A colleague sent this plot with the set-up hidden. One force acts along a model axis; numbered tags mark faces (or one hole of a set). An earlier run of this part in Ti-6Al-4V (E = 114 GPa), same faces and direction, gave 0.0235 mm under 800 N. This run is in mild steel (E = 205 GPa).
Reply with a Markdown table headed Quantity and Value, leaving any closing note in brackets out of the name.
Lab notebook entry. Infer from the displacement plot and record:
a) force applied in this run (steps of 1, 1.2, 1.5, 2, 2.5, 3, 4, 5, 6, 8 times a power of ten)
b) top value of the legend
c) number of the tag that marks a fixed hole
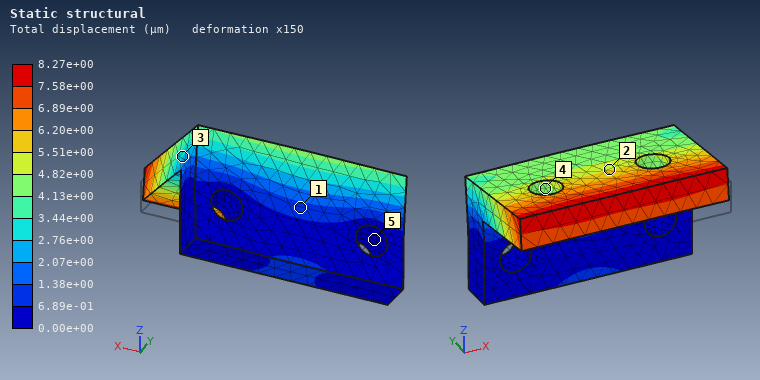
| Quantity | Value |
|---|---|
| force applied in this run | 500 N |
| top value of the legend | 8.27e+00 µm |
| number of the tag that marks a fixed hole | 5 |
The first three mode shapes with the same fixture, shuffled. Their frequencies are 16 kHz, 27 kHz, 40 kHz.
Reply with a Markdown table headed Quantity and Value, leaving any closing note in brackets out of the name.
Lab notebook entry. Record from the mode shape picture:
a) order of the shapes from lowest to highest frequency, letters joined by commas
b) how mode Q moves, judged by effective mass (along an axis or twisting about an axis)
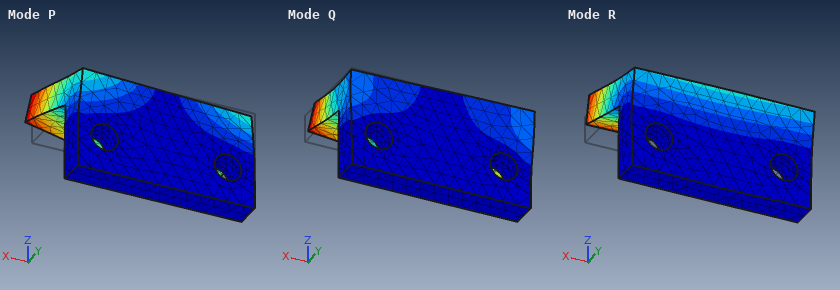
| Quantity | Value |
|---|---|
| order of the shapes from lowest to highest frequency, letters joined by commas | R, P, Q |
| how mode Q moves, judged by effective mass | along X |
